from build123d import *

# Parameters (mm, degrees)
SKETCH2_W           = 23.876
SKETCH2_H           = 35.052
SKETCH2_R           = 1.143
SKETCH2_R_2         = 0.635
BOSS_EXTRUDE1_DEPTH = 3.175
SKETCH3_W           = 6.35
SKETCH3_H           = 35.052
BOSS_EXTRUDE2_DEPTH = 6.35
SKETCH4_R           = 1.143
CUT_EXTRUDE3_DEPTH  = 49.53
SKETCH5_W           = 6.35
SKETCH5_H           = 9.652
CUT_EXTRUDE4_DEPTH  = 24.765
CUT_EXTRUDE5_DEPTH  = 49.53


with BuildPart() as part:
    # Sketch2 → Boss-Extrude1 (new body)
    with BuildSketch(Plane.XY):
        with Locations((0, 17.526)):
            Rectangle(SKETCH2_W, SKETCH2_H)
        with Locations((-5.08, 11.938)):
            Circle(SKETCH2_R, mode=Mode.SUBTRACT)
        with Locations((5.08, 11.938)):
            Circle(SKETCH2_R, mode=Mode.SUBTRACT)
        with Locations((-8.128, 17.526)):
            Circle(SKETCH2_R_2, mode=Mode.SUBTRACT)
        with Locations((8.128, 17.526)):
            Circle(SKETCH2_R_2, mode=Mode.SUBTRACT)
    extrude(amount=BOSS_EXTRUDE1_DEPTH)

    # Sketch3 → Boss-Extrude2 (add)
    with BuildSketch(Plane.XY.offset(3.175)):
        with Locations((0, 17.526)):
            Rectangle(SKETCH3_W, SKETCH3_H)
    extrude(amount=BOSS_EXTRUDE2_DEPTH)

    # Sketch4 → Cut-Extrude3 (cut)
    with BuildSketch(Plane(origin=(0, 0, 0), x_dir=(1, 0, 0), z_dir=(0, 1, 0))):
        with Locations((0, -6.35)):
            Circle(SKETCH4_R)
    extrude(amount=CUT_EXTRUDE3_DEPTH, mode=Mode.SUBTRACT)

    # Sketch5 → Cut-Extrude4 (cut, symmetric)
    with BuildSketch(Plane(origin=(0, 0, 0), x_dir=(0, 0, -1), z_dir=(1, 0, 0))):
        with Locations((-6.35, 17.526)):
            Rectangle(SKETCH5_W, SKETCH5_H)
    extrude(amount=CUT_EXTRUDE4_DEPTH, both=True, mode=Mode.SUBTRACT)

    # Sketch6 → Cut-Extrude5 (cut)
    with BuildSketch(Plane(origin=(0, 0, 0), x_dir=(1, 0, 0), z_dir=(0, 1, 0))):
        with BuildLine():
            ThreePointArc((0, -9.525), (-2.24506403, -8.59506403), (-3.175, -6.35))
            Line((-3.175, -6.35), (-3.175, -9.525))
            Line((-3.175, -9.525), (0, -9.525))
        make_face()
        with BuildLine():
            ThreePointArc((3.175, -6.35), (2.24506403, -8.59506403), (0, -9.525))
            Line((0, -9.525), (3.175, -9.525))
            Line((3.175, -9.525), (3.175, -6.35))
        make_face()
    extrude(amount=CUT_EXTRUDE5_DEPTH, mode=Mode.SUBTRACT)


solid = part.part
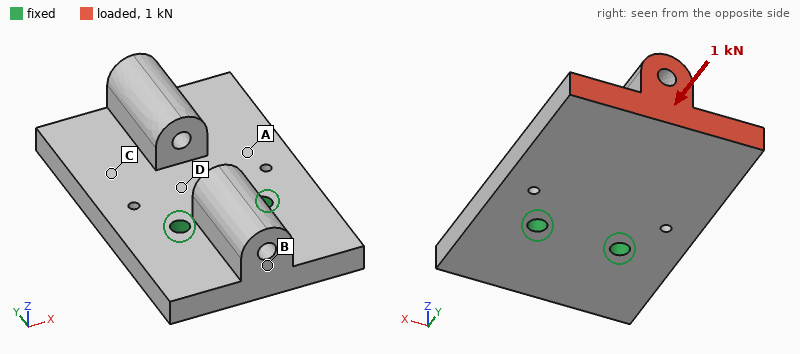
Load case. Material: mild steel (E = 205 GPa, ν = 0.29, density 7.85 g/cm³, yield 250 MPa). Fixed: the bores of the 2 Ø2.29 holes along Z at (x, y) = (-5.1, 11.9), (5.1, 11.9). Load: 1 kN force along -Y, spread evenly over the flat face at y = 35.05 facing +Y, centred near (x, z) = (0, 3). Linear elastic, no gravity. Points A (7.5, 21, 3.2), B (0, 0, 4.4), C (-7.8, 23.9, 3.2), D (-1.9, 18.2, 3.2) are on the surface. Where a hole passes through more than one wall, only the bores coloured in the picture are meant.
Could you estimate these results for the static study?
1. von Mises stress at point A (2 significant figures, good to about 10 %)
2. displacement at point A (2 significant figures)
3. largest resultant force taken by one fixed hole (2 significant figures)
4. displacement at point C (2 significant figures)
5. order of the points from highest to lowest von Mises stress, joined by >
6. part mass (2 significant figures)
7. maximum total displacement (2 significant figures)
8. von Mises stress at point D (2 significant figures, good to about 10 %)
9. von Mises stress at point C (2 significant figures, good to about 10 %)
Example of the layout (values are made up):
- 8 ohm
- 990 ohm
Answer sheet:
- 37 MPa
- 5.0 µm
- 500 N
- 8.1 µm
- D > A > C > B
- 27 g
- 26 µm
- 48 MPa
- 30 MPa
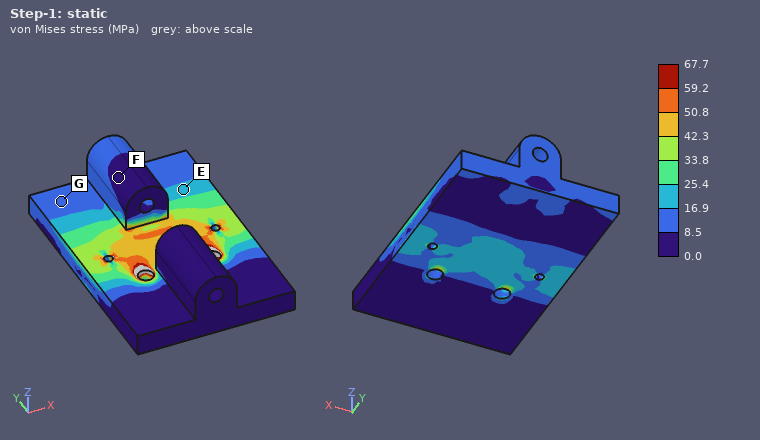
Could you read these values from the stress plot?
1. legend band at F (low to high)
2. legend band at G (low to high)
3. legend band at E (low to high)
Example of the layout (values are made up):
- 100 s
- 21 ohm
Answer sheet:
- 0.0 to 8.5 MPa
- 8.5 to 16.9 MPa
- 16.9 to 25.4 MPa
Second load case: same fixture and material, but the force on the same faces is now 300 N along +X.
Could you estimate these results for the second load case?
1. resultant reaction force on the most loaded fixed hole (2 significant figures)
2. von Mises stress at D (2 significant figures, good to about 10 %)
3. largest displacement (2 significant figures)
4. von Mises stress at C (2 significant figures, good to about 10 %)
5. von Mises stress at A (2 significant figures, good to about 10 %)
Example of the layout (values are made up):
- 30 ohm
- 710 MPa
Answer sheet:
- 620 N
- 21 MPa
- 6.3 µm
- 12 MPa
- 12 MPa
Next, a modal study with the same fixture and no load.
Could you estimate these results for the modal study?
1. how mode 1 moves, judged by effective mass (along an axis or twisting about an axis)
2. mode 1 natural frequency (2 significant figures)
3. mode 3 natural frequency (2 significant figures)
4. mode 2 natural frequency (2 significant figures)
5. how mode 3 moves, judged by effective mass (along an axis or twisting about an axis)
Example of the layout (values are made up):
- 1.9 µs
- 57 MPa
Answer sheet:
- along Z
- 3900 Hz
- 15 kHz
- 10 kHz
- along Z
